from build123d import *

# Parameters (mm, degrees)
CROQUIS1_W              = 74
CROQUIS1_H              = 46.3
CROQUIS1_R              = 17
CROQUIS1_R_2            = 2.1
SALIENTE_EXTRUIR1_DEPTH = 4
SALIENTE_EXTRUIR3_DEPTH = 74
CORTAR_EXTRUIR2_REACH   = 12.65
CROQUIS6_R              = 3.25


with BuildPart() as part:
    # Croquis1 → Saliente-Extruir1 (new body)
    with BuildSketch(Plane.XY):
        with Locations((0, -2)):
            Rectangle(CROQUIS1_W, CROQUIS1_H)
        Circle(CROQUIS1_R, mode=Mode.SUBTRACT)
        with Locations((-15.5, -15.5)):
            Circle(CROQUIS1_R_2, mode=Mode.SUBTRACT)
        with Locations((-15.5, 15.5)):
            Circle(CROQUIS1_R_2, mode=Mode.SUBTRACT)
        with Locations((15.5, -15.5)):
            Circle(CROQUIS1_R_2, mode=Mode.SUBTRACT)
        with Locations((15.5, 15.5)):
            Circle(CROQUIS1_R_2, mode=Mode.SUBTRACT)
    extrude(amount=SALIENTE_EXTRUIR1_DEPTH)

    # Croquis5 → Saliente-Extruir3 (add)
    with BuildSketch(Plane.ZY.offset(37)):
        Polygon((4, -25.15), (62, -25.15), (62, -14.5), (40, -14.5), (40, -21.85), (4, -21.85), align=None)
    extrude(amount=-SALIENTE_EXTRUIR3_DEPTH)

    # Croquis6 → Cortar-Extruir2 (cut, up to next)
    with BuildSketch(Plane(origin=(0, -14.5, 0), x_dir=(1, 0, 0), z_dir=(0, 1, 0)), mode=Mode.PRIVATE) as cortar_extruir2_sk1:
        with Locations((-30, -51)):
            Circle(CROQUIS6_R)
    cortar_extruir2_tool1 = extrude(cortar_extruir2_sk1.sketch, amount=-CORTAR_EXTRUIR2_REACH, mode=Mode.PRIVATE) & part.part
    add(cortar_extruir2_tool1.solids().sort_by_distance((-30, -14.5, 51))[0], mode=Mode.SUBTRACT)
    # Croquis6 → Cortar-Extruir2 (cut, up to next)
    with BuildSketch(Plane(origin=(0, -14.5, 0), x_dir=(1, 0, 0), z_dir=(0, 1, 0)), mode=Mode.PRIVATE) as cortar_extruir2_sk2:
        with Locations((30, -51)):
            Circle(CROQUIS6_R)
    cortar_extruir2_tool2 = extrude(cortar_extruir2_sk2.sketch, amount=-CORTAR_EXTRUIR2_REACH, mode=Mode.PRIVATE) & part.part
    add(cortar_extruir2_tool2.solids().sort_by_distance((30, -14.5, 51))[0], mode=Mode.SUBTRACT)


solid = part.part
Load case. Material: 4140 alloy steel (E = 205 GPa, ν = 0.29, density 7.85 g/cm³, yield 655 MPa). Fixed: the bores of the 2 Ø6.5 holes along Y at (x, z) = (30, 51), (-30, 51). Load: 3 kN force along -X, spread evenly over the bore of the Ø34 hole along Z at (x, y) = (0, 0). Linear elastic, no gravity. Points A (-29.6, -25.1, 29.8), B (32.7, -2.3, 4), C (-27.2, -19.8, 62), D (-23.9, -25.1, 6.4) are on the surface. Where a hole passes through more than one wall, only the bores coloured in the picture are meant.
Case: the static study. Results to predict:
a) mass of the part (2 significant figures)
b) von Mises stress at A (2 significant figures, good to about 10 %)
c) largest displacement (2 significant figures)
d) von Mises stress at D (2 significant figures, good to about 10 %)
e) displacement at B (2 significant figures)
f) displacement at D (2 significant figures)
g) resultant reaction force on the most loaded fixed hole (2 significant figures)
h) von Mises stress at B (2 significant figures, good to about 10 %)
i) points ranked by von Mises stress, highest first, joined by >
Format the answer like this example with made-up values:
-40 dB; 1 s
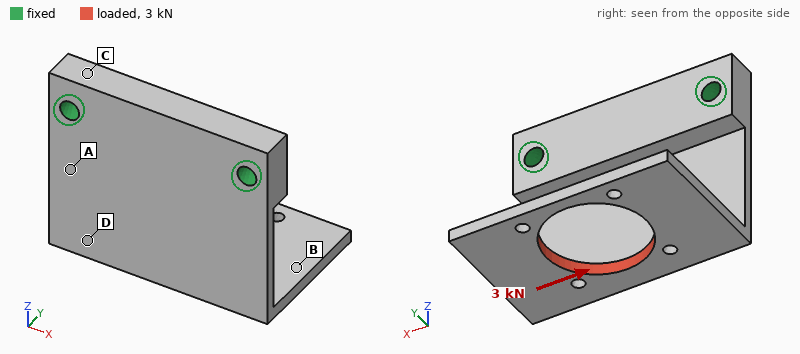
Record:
280 g; 280 MPa; 1.0 mm; 220 MPa; 0.67 mm; 0.35 mm; 3.0 kN; 100 MPa; A > D > B > C
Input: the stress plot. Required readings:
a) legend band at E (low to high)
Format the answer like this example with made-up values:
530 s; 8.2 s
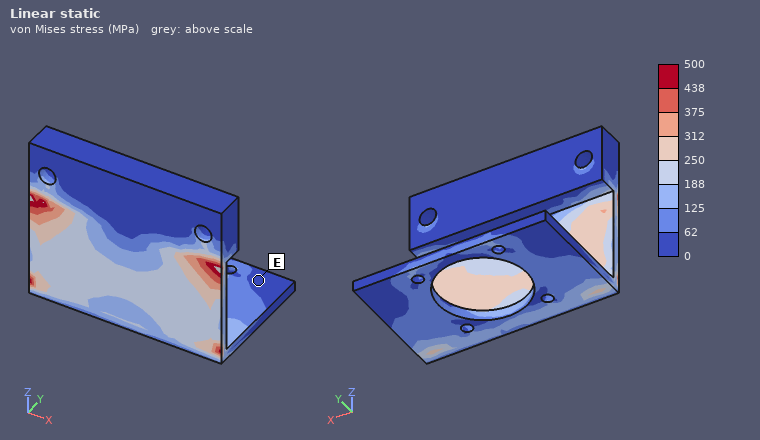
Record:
0 to 62 MPa
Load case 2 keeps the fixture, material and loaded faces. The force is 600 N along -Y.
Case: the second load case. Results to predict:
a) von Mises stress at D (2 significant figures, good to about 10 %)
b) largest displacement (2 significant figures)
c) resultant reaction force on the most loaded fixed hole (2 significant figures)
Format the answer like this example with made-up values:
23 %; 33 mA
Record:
19 MPa; 0.53 mm; 300 N
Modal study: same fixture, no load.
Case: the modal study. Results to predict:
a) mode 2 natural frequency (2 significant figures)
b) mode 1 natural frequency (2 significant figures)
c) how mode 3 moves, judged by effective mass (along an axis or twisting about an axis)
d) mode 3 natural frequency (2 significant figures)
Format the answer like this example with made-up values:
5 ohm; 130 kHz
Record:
980 Hz; 560 Hz; along Y; 1500 Hz
